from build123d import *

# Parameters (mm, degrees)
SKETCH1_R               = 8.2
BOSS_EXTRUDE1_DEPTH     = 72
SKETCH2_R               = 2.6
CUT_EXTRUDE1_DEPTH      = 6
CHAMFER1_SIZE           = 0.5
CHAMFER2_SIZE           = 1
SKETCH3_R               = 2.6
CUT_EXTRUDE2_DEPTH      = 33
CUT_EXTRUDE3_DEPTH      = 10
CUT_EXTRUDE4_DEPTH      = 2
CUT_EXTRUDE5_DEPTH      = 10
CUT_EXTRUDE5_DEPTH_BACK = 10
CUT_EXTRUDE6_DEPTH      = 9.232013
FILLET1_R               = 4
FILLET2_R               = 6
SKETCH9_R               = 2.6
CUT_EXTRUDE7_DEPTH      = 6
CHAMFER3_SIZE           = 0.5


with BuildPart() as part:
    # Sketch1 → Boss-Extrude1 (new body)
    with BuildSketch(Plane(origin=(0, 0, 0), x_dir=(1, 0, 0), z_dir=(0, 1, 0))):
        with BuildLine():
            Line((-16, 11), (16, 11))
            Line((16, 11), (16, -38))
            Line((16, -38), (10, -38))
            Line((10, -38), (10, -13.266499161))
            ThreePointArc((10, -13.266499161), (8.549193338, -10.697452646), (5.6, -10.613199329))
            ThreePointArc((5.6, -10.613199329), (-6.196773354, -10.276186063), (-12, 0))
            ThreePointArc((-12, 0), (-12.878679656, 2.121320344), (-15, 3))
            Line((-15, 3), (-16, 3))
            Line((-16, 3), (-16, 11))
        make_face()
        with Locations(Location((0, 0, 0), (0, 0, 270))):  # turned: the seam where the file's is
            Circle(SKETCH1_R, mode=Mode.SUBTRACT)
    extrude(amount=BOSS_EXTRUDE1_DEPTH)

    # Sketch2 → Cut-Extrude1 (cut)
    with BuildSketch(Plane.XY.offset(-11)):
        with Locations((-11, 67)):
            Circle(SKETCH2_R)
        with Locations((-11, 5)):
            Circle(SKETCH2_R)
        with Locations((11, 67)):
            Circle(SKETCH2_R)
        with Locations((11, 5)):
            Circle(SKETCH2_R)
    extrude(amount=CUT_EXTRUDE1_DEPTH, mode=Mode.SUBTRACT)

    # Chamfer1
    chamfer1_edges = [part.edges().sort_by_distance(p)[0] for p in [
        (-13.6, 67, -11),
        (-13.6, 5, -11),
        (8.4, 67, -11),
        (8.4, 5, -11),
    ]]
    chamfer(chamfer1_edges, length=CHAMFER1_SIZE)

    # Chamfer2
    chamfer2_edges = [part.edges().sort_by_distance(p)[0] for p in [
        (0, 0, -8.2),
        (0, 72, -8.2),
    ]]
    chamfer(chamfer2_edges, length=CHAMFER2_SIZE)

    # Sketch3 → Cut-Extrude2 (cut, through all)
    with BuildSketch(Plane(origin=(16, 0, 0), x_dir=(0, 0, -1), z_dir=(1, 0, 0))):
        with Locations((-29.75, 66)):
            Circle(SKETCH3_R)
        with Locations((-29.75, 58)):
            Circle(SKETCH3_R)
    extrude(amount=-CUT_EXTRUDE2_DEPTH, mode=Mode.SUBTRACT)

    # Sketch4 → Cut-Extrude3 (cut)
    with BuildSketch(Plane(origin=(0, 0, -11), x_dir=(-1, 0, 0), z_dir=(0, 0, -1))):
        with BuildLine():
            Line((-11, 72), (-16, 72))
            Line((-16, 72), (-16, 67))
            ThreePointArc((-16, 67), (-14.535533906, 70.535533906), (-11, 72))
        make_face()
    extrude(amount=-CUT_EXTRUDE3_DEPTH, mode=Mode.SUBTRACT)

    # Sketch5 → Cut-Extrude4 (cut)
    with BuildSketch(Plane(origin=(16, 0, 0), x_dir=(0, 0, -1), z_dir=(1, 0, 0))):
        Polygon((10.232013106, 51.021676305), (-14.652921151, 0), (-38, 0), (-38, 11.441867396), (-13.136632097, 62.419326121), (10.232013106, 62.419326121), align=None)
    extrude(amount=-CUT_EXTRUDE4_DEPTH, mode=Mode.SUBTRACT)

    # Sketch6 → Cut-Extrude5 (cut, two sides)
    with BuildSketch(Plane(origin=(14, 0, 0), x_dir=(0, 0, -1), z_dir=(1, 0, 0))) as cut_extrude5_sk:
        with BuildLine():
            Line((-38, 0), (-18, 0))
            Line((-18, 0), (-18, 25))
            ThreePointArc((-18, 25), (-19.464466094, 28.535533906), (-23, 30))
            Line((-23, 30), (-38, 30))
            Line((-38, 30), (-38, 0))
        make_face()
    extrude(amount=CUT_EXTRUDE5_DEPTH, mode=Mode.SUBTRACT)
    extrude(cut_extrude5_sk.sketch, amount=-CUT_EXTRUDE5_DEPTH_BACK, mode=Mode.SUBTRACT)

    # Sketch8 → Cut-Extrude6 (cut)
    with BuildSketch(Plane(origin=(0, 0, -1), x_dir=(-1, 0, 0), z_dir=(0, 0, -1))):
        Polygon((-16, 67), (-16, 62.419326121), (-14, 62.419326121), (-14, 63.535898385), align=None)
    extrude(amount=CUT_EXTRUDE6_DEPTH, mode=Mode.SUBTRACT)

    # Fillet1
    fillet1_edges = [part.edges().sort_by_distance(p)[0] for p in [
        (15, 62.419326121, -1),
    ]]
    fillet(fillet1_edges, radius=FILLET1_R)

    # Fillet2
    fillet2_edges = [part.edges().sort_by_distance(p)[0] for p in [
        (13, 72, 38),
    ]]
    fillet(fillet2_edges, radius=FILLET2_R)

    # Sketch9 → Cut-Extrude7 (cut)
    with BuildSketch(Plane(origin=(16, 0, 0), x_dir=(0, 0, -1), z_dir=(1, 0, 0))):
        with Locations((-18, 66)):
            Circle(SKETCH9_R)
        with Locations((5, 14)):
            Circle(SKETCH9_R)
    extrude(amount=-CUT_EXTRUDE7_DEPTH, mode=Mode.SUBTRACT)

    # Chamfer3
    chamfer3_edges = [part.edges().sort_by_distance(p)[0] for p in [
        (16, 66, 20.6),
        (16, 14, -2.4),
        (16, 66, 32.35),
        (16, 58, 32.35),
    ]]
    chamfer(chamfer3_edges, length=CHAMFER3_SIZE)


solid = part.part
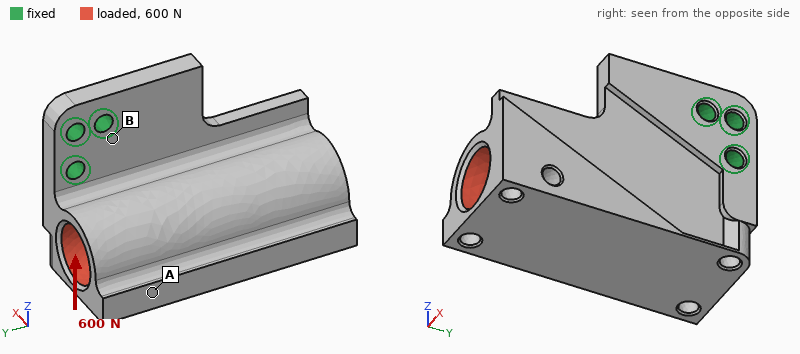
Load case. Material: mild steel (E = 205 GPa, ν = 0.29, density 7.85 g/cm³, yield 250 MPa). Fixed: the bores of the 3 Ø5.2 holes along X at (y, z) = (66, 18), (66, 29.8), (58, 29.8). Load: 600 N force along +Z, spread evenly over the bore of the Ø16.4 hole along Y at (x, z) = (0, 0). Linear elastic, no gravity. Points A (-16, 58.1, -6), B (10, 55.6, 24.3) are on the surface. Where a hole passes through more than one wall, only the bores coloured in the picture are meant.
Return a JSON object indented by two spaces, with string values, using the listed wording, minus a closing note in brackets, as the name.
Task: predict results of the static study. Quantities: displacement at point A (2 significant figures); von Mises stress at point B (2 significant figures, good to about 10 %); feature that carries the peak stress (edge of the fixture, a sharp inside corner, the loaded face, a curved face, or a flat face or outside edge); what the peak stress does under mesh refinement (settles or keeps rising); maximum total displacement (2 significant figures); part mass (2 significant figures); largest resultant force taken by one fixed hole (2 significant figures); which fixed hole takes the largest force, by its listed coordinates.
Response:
{
  "displacement at point A": "35 µm",
  "von Mises stress at point B": "25 MPa",
  "feature that carries the peak stress": "edge of the fixture",
  "what the peak stress does under mesh refinement": "keeps rising",
  "maximum total displacement": "52 µm",
  "part mass": "270 g",
  "largest resultant force taken by one fixed hole": "950 N",
  "which fixed hole takes the largest force, by its listed coordinates": "(58, 29.8)"
}
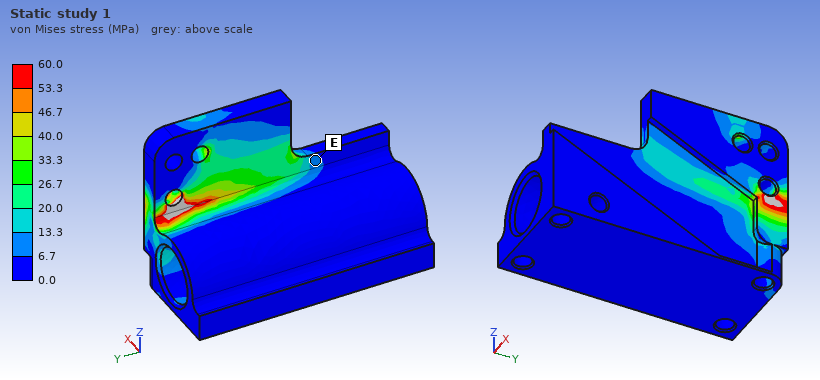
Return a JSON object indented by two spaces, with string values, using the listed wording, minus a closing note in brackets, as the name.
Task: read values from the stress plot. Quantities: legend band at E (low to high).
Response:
{
  "legend band at E": "6.7 to 13.3 MPa"
}
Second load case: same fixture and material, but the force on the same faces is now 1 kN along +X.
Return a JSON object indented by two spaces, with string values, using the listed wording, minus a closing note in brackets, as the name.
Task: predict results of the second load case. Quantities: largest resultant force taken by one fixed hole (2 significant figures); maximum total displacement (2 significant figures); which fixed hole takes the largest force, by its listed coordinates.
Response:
{
  "largest resultant force taken by one fixed hole": "760 N",
  "maximum total displacement": "0.21 mm",
  "which fixed hole takes the largest force, by its listed coordinates": "(66, 18)"
}
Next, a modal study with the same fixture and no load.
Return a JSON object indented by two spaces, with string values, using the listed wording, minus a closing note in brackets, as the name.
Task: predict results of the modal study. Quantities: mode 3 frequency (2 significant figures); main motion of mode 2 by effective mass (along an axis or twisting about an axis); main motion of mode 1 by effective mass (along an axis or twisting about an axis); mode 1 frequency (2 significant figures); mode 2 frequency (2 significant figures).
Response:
{
  "mode 3 frequency": "3400 Hz",
  "main motion of mode 2 by effective mass": "along Z",
  "main motion of mode 1 by effective mass": "along X",
  "mode 1 frequency": "890 Hz",
  "mode 2 frequency": "2000 Hz"
}
